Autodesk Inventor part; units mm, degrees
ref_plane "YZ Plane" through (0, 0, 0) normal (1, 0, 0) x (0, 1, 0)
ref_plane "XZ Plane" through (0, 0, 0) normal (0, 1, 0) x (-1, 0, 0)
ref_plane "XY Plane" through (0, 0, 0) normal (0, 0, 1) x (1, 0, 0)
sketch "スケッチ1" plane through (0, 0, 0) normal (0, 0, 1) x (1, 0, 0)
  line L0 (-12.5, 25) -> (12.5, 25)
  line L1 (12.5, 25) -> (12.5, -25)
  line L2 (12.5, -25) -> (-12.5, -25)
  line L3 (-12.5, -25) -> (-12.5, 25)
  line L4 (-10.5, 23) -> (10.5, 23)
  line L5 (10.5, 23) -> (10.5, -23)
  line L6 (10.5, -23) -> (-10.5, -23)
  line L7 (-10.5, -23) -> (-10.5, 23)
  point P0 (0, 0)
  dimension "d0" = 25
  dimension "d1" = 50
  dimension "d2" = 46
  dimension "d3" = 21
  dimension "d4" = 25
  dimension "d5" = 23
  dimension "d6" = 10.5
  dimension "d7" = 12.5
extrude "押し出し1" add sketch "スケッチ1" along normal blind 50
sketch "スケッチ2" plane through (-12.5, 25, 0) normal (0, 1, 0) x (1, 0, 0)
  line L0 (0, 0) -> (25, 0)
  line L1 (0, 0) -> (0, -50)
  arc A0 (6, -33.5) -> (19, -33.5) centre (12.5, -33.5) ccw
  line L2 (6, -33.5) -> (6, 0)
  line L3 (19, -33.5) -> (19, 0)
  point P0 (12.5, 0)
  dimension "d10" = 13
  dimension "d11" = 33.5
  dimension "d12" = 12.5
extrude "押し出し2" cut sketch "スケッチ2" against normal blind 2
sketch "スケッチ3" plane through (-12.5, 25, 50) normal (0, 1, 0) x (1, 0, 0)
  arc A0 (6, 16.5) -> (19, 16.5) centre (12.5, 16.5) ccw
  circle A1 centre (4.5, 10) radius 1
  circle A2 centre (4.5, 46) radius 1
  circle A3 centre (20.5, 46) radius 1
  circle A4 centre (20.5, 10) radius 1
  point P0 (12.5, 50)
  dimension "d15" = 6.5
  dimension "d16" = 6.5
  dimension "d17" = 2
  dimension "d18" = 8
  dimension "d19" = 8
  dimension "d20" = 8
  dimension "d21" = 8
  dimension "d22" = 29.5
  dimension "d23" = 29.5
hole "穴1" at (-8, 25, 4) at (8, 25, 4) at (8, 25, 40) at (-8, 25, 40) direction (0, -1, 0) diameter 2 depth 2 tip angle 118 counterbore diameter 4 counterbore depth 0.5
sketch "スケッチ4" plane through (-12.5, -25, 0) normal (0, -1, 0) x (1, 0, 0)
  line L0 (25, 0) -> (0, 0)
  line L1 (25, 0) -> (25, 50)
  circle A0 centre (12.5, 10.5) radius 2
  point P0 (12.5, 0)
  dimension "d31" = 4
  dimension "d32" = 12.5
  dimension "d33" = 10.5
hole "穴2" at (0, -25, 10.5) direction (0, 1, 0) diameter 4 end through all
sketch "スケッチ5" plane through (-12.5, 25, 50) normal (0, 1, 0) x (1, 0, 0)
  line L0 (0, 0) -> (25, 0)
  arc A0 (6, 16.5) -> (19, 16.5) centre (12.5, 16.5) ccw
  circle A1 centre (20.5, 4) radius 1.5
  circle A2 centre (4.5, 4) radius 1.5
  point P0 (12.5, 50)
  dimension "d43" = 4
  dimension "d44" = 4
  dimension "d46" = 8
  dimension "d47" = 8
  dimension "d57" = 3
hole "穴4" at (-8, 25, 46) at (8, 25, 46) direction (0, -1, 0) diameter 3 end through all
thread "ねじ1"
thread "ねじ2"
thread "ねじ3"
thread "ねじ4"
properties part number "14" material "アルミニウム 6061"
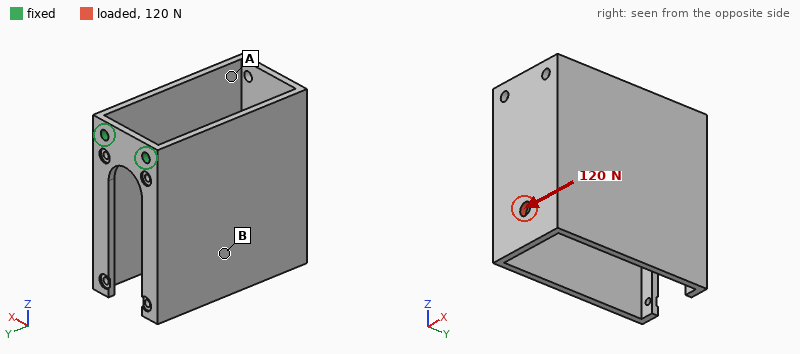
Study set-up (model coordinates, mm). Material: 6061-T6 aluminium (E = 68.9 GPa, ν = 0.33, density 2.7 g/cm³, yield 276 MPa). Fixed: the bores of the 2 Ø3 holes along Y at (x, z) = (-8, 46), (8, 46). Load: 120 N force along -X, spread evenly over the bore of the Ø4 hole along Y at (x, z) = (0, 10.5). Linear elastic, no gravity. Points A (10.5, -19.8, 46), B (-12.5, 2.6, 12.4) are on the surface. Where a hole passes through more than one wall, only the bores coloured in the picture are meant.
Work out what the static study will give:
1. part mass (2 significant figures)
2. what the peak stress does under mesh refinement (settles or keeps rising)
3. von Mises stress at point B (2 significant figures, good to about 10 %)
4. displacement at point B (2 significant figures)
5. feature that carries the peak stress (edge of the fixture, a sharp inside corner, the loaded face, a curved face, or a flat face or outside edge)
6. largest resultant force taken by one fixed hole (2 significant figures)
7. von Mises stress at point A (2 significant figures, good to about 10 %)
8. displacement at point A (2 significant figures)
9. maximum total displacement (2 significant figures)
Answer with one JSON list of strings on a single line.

["35 g", "keeps rising", "11 MPa", "0.35 mm", "edge of the fixture", "290 N", "40 MPa", "0.49 mm", "0.63 mm"]
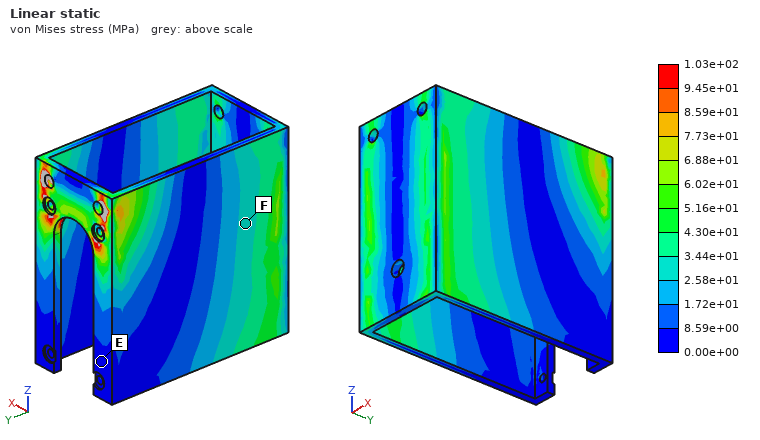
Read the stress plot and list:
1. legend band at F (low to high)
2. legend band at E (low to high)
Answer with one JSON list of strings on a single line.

["2.58e+01 to 3.44e+01 MPa", "0.00e+00 to 8.59e+00 MPa"]
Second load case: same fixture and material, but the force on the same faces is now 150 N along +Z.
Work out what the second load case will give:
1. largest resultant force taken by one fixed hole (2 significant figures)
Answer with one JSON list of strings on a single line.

["76 N"]
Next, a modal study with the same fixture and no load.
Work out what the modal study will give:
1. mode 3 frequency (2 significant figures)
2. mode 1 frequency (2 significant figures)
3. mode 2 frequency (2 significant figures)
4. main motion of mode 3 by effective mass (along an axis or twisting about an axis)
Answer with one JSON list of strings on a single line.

["1100 Hz", "550 Hz", "560 Hz", "twisting about Y"]
